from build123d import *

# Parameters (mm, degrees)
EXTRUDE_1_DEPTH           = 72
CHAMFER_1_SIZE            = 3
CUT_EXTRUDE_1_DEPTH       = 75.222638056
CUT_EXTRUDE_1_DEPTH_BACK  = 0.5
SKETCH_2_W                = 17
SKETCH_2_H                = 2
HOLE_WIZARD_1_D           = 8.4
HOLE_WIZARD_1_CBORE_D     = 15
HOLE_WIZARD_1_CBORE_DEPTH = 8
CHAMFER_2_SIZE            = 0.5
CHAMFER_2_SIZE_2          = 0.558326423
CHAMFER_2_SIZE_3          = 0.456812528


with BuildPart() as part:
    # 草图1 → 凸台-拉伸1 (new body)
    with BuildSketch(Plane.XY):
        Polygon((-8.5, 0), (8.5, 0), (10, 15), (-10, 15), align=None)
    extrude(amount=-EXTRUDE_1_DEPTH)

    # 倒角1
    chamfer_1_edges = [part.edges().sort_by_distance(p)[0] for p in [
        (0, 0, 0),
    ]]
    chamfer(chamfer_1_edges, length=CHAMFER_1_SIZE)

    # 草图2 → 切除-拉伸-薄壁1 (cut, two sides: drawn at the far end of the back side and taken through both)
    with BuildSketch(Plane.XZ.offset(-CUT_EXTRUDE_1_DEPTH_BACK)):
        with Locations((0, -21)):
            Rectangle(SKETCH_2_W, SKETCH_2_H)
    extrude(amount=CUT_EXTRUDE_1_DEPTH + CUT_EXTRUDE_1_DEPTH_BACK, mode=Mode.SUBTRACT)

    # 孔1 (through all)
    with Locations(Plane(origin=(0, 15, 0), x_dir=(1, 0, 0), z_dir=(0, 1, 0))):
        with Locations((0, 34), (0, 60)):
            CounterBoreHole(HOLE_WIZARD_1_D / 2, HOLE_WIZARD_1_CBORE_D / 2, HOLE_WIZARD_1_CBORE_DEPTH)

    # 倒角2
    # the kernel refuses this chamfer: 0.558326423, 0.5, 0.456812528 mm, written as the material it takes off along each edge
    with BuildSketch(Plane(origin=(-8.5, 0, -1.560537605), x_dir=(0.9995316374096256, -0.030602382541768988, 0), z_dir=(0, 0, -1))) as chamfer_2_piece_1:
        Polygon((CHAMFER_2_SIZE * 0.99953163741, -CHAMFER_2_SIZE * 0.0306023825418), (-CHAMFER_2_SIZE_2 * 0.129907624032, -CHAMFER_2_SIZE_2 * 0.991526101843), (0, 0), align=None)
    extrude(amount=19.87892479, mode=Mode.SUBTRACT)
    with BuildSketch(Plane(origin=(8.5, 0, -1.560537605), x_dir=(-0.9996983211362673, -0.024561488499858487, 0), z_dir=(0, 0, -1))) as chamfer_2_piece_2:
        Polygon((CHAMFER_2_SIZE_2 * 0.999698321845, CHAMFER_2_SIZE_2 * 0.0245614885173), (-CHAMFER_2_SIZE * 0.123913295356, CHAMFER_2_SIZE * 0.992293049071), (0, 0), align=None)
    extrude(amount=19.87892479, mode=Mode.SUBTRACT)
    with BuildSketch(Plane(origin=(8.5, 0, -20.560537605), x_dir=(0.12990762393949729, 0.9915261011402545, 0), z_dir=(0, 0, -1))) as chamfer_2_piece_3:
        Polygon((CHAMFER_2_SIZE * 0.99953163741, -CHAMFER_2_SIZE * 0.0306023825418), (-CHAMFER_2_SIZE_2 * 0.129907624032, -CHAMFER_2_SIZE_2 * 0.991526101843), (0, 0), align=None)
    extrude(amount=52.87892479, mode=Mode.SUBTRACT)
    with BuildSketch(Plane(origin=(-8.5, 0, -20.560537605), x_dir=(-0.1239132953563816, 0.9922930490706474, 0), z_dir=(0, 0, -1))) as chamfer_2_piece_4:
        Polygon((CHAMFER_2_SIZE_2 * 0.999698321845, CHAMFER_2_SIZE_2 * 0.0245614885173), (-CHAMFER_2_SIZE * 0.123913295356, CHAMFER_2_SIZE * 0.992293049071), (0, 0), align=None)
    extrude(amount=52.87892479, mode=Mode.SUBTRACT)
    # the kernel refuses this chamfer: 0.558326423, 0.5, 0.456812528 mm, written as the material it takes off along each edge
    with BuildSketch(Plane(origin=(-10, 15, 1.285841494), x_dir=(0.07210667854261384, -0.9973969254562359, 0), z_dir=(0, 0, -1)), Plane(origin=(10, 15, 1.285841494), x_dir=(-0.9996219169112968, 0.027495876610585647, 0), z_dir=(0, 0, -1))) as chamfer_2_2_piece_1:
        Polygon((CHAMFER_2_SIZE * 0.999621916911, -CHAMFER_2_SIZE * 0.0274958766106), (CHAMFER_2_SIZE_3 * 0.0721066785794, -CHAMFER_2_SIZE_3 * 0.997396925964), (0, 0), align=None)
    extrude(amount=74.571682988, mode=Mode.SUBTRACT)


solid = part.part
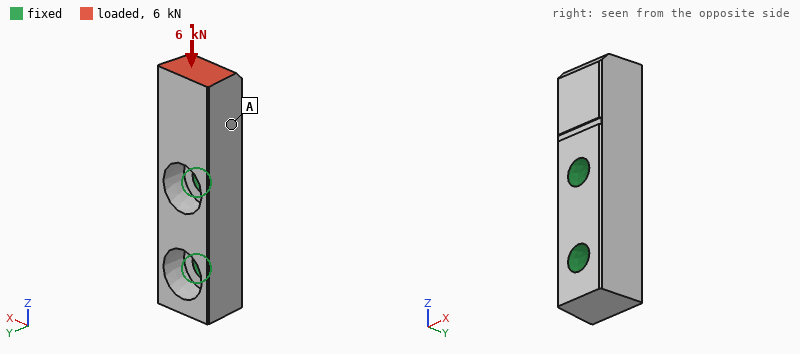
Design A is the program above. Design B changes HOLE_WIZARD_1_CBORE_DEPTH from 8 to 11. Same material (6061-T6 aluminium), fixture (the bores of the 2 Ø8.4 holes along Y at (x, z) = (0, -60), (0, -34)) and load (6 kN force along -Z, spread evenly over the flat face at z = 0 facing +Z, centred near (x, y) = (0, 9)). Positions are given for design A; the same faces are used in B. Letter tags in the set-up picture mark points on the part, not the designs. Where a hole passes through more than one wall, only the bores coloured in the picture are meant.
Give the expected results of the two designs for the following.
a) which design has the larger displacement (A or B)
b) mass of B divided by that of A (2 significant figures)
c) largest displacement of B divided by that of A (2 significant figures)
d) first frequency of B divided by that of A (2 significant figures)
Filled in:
B
0.96
1.5
0.86
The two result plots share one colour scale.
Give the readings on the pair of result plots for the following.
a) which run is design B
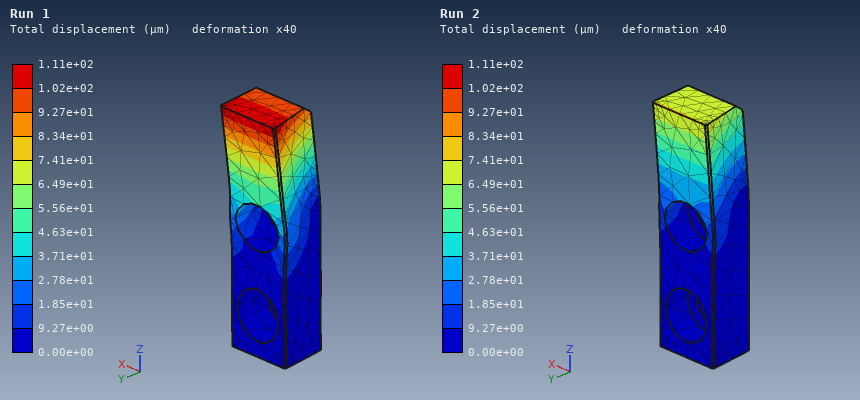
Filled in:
Run 1
